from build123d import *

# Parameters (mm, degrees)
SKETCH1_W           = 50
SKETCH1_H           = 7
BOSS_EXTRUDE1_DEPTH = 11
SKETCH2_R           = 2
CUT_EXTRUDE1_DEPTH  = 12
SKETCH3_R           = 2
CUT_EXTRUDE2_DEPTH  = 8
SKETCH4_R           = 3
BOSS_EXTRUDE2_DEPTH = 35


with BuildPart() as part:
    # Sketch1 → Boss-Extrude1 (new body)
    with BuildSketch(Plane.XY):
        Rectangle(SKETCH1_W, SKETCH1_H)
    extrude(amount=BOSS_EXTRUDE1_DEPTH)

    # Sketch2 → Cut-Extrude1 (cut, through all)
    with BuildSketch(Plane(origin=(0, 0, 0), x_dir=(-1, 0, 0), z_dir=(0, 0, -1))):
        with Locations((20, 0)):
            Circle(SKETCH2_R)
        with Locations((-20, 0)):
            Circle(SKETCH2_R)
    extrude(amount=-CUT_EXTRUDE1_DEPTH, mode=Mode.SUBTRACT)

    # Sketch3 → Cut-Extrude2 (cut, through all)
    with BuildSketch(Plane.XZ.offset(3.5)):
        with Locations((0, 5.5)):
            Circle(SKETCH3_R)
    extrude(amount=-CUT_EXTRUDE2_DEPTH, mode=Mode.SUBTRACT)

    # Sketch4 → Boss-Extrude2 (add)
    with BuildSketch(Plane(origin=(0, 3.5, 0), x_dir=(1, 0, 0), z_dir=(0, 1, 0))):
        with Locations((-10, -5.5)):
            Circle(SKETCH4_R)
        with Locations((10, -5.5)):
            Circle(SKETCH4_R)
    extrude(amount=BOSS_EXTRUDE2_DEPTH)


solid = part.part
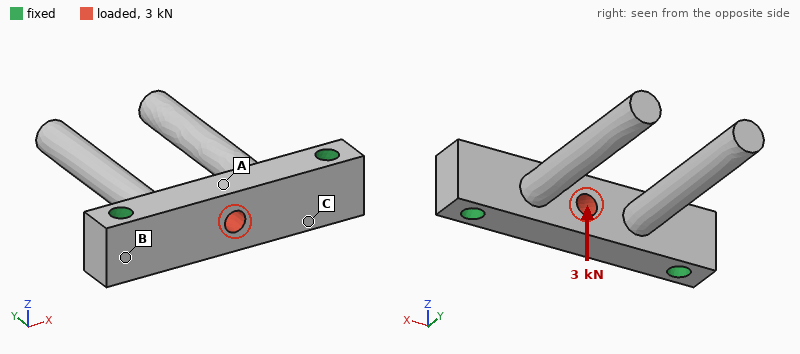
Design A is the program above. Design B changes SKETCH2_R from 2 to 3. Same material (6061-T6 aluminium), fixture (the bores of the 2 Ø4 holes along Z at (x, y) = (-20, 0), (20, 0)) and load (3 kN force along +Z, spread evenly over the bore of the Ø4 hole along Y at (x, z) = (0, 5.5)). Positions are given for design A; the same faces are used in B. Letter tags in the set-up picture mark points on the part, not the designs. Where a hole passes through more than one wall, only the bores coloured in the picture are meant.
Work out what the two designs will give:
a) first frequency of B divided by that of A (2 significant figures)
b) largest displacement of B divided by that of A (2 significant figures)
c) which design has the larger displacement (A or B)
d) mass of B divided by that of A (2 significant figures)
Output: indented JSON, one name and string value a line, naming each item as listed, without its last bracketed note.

{
  "first frequency of B divided by that of A": "1.0",
  "largest displacement of B divided by that of A": "0.87",
  "which design has the larger displacement": "A",
  "mass of B divided by that of A": "0.94"
}
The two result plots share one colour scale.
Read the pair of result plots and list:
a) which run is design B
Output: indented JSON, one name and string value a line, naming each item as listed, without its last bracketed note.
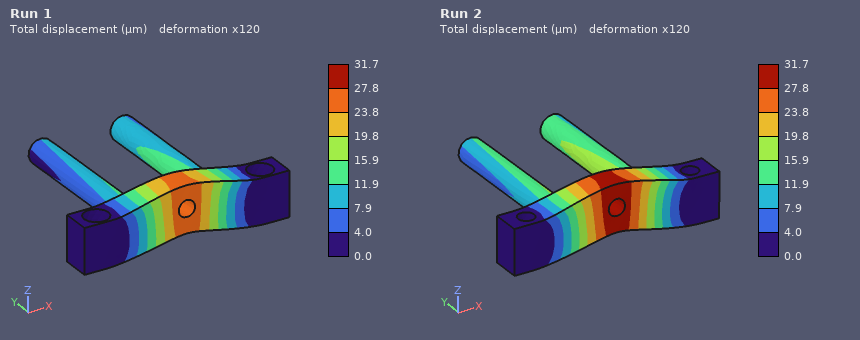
{
  "which run is design B": "Run 1"
}
